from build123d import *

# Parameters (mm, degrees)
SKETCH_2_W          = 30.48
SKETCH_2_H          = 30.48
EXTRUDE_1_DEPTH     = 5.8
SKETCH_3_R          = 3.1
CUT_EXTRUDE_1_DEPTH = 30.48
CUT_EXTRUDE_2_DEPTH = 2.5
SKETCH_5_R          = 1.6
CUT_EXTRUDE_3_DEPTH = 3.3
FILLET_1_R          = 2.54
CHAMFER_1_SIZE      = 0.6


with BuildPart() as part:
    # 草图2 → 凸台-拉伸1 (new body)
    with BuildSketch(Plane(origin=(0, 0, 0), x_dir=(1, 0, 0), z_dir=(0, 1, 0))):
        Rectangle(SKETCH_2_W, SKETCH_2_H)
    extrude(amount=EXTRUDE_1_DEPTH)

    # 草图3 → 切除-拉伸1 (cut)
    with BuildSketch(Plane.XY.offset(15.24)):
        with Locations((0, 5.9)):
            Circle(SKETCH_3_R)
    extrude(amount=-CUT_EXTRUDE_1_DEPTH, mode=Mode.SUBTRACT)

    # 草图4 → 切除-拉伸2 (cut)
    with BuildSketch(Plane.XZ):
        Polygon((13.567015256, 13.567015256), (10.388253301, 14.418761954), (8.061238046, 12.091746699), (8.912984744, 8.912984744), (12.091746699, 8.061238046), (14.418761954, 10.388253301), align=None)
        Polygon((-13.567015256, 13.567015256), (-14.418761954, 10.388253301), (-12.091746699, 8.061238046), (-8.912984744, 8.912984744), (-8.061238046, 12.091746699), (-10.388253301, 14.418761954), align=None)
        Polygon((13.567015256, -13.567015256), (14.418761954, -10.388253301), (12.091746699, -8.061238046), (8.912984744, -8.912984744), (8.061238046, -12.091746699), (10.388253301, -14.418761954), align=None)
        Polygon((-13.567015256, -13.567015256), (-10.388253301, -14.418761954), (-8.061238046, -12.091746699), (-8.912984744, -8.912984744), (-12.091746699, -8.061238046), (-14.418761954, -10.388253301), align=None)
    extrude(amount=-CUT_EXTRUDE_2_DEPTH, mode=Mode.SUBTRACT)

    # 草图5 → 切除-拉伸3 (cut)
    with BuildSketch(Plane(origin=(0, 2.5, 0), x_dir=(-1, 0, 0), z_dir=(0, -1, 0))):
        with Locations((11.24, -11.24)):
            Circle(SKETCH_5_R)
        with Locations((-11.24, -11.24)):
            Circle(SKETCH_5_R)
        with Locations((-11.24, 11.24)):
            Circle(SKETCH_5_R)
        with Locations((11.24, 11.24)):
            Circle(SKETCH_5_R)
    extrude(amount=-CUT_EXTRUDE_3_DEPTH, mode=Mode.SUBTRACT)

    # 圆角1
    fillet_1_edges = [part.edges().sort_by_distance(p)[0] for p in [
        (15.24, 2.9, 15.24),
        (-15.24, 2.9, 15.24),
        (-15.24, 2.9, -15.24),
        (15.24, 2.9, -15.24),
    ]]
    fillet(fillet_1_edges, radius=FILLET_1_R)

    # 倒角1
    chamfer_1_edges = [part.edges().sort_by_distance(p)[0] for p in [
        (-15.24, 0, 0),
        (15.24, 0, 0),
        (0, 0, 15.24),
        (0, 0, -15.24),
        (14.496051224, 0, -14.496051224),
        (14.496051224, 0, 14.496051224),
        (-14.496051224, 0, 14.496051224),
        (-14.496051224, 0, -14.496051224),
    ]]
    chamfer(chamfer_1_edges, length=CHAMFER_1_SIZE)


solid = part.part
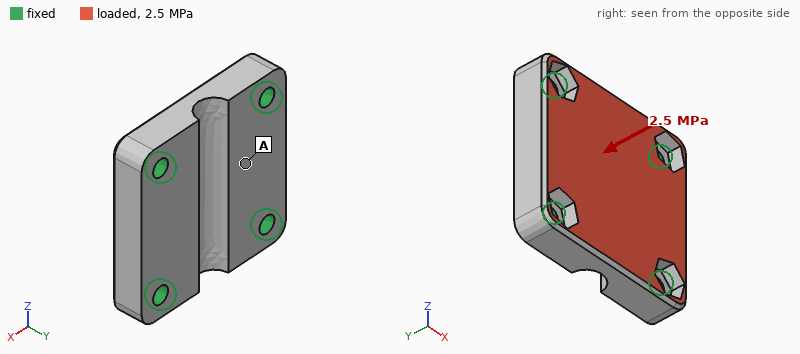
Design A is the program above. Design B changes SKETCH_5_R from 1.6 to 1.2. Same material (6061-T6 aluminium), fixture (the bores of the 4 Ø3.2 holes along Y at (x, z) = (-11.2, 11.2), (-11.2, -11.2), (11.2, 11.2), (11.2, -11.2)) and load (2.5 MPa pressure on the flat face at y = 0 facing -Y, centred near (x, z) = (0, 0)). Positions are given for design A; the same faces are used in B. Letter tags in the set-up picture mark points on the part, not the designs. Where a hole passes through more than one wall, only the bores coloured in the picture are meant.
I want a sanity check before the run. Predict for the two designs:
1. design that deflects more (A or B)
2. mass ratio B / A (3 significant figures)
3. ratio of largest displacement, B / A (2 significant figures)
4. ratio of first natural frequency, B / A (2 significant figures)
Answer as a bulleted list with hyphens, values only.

- B
- 1.01
- 1.2
- 0.91
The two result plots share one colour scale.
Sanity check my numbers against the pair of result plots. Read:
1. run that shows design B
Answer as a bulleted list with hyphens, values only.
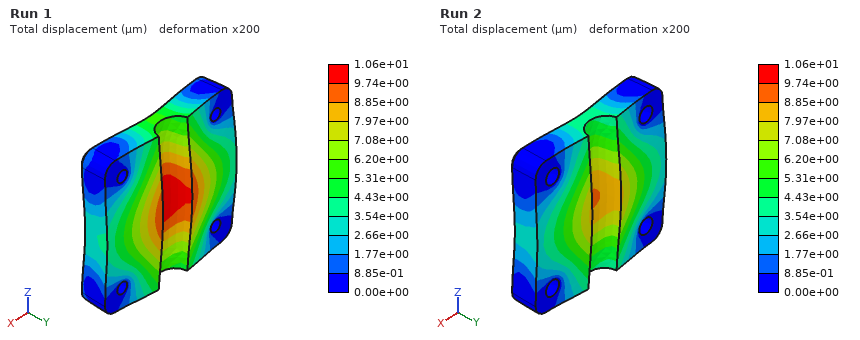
- Run 1
